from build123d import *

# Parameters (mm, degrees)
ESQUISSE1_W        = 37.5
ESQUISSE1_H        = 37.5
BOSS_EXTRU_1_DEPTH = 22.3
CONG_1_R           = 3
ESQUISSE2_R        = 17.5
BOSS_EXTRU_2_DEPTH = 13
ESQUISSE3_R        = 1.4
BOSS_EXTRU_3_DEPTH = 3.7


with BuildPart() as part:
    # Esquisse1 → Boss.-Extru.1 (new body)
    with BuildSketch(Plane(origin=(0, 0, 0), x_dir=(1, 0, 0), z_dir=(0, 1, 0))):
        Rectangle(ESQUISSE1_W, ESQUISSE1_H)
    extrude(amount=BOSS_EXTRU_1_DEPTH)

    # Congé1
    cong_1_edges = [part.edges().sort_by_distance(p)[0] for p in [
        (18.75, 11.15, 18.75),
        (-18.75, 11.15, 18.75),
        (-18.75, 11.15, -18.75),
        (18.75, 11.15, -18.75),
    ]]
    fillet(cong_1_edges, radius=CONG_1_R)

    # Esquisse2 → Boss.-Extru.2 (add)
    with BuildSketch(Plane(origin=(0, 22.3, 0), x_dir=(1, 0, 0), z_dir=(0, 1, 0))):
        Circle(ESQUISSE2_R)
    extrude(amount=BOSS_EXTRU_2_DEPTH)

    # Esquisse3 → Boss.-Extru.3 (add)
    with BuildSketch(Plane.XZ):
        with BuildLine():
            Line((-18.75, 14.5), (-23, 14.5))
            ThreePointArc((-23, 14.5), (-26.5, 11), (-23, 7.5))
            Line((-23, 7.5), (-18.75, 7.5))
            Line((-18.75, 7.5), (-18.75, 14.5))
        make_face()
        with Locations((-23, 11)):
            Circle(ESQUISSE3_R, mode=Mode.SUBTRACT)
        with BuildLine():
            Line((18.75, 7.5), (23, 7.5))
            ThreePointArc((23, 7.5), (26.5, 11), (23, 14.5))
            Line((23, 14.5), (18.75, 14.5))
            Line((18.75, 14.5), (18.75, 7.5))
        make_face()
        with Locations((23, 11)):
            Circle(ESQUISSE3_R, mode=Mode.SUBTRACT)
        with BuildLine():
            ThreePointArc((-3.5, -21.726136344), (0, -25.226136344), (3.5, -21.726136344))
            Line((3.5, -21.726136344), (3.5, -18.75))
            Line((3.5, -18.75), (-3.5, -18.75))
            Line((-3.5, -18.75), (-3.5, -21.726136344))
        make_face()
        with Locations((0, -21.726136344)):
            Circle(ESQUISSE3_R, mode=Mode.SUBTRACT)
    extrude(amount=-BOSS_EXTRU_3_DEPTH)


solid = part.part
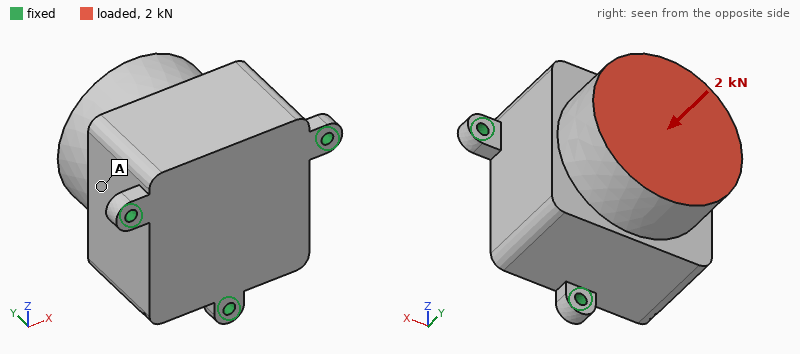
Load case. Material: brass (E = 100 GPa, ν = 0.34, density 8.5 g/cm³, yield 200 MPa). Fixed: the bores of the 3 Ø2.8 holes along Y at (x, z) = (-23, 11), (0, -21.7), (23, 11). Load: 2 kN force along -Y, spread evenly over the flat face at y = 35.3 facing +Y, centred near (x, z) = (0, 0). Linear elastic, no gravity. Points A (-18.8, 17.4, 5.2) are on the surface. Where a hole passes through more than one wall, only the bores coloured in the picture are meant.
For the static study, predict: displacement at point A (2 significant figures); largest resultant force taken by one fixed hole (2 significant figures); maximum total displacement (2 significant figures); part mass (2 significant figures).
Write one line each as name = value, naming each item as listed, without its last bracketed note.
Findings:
displacement at point A = 6.7 µm
largest resultant force taken by one fixed hole = 750 N
maximum total displacement = 8.0 µm
part mass = 380 g
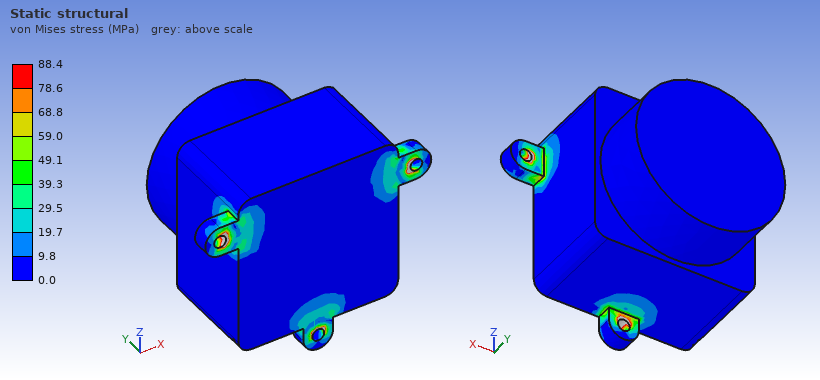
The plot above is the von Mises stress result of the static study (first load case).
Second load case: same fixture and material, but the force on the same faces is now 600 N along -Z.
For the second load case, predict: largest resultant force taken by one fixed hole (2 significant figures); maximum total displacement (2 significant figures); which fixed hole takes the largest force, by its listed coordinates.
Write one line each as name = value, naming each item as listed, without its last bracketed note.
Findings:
largest resultant force taken by one fixed hole = 790 N
maximum total displacement = 11 µm
which fixed hole takes the largest force, by its listed coordinates = (0, -21.7)
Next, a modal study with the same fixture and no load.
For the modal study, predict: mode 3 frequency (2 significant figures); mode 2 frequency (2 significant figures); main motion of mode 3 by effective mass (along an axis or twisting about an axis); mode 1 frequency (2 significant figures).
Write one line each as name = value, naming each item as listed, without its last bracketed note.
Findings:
mode 3 frequency = 4800 Hz
mode 2 frequency = 3400 Hz
main motion of mode 3 by effective mass = along Y
mode 1 frequency = 3300 Hz
